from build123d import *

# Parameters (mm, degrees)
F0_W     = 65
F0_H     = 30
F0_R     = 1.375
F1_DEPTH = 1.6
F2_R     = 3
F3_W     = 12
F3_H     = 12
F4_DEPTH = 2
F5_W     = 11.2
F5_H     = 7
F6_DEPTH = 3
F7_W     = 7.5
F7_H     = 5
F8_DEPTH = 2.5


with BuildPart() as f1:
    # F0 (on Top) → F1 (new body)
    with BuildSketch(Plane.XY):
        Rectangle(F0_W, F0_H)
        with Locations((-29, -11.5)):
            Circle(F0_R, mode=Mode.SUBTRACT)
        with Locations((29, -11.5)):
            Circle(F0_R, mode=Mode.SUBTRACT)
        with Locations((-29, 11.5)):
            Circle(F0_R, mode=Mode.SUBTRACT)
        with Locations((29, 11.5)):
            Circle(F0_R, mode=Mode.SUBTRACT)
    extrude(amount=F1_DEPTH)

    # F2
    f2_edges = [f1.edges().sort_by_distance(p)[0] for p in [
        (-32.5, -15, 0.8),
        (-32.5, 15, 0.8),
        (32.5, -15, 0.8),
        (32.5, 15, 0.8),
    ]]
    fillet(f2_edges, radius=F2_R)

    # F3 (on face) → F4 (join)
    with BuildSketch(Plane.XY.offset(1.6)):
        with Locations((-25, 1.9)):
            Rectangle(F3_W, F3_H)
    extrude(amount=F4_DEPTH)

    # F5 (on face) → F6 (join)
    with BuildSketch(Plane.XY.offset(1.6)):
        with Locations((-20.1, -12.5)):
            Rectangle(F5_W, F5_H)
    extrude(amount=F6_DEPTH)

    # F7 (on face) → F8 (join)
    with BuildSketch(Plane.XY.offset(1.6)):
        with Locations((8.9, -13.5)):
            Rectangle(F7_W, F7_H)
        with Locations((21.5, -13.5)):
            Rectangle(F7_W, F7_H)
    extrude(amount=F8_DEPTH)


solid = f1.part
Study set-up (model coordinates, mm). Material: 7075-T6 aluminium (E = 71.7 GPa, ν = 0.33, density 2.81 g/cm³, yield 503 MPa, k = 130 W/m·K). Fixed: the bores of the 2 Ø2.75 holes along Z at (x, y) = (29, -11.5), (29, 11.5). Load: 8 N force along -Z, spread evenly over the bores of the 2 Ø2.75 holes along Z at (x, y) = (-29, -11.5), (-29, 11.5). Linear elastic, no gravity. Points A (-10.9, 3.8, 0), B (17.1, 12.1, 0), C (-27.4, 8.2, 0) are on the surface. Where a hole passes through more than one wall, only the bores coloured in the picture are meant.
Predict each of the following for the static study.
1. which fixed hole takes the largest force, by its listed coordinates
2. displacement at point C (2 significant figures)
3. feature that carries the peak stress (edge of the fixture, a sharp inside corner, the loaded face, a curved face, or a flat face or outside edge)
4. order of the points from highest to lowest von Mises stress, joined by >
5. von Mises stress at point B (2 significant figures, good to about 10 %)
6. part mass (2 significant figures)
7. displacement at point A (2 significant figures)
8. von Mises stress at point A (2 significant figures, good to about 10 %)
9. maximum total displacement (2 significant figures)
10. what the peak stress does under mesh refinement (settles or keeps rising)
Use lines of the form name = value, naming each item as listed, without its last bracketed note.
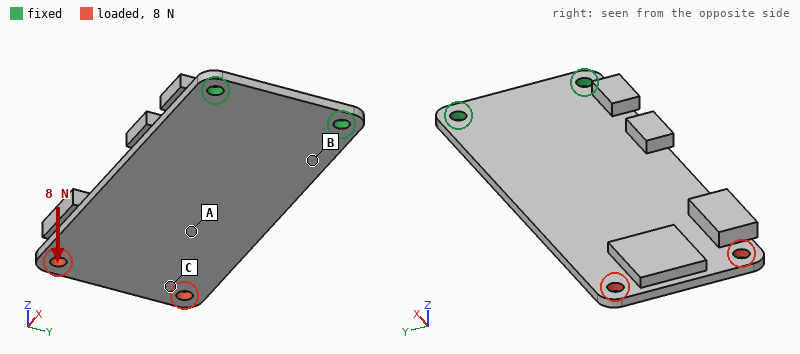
which fixed hole takes the largest force, by its listed coordinates = (29, -11.5)
displacement at point C = 0.61 mm
feature that carries the peak stress = edge of the fixture
order of the points from highest to lowest von Mises stress, joined by > = B > A > C
von Mises stress at point B = 25 MPa
part mass = 11 g
displacement at point A = 0.35 mm
von Mises stress at point A = 10 MPa
maximum total displacement = 0.70 mm
what the peak stress does under mesh refinement = keeps rising
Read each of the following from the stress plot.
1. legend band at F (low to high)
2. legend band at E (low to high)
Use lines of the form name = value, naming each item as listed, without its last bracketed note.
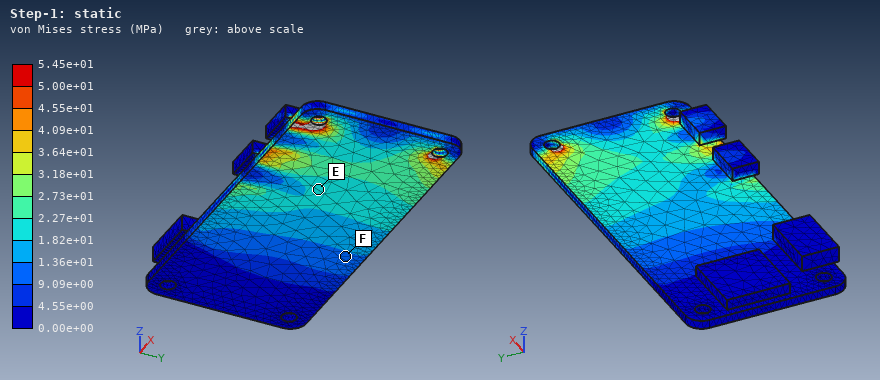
legend band at F = 9.09e+00 to 1.36e+01 MPa
legend band at E = 1.82e+01 to 2.27e+01 MPa
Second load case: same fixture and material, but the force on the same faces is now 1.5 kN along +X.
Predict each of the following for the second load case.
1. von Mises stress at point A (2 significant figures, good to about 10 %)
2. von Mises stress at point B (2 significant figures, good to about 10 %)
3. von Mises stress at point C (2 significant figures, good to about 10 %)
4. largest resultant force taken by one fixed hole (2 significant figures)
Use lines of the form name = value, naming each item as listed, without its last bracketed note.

von Mises stress at point A = 29 MPa
von Mises stress at point B = 40 MPa
von Mises stress at point C = 55 MPa
largest resultant force taken by one fixed hole = 770 N
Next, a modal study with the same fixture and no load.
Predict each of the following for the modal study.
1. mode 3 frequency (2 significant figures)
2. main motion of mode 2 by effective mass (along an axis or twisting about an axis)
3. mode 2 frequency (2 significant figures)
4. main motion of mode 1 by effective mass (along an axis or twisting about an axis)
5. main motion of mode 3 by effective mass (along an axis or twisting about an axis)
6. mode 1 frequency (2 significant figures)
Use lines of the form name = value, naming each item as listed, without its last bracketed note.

mode 3 frequency = 2100 Hz
main motion of mode 2 by effective mass = twisting about X
mode 2 frequency = 1400 Hz
main motion of mode 1 by effective mass = along Z
main motion of mode 3 by effective mass = along Z
mode 1 frequency = 310 Hz
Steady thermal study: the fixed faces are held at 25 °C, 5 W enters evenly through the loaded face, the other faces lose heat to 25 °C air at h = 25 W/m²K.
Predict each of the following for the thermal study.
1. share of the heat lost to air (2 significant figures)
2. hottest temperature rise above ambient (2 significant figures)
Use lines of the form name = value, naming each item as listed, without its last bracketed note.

share of the heat lost to air = 37 %
hottest temperature rise above ambient = 37 K
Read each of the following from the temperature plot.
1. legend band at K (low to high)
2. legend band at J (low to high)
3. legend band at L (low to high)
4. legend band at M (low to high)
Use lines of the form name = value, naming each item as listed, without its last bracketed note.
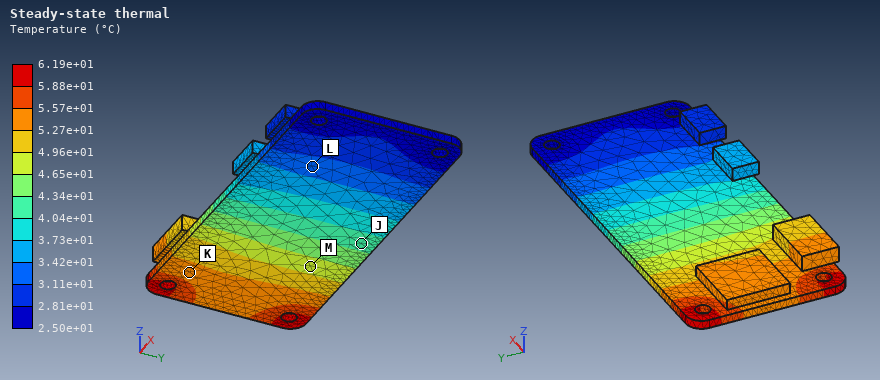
legend band at K = 5.27e+01 to 5.57e+01 °C
legend band at J = 4.04e+01 to 4.34e+01 °C
legend band at L = 3.11e+01 to 3.42e+01 °C
legend band at M = 4.65e+01 to 4.96e+01 °C
